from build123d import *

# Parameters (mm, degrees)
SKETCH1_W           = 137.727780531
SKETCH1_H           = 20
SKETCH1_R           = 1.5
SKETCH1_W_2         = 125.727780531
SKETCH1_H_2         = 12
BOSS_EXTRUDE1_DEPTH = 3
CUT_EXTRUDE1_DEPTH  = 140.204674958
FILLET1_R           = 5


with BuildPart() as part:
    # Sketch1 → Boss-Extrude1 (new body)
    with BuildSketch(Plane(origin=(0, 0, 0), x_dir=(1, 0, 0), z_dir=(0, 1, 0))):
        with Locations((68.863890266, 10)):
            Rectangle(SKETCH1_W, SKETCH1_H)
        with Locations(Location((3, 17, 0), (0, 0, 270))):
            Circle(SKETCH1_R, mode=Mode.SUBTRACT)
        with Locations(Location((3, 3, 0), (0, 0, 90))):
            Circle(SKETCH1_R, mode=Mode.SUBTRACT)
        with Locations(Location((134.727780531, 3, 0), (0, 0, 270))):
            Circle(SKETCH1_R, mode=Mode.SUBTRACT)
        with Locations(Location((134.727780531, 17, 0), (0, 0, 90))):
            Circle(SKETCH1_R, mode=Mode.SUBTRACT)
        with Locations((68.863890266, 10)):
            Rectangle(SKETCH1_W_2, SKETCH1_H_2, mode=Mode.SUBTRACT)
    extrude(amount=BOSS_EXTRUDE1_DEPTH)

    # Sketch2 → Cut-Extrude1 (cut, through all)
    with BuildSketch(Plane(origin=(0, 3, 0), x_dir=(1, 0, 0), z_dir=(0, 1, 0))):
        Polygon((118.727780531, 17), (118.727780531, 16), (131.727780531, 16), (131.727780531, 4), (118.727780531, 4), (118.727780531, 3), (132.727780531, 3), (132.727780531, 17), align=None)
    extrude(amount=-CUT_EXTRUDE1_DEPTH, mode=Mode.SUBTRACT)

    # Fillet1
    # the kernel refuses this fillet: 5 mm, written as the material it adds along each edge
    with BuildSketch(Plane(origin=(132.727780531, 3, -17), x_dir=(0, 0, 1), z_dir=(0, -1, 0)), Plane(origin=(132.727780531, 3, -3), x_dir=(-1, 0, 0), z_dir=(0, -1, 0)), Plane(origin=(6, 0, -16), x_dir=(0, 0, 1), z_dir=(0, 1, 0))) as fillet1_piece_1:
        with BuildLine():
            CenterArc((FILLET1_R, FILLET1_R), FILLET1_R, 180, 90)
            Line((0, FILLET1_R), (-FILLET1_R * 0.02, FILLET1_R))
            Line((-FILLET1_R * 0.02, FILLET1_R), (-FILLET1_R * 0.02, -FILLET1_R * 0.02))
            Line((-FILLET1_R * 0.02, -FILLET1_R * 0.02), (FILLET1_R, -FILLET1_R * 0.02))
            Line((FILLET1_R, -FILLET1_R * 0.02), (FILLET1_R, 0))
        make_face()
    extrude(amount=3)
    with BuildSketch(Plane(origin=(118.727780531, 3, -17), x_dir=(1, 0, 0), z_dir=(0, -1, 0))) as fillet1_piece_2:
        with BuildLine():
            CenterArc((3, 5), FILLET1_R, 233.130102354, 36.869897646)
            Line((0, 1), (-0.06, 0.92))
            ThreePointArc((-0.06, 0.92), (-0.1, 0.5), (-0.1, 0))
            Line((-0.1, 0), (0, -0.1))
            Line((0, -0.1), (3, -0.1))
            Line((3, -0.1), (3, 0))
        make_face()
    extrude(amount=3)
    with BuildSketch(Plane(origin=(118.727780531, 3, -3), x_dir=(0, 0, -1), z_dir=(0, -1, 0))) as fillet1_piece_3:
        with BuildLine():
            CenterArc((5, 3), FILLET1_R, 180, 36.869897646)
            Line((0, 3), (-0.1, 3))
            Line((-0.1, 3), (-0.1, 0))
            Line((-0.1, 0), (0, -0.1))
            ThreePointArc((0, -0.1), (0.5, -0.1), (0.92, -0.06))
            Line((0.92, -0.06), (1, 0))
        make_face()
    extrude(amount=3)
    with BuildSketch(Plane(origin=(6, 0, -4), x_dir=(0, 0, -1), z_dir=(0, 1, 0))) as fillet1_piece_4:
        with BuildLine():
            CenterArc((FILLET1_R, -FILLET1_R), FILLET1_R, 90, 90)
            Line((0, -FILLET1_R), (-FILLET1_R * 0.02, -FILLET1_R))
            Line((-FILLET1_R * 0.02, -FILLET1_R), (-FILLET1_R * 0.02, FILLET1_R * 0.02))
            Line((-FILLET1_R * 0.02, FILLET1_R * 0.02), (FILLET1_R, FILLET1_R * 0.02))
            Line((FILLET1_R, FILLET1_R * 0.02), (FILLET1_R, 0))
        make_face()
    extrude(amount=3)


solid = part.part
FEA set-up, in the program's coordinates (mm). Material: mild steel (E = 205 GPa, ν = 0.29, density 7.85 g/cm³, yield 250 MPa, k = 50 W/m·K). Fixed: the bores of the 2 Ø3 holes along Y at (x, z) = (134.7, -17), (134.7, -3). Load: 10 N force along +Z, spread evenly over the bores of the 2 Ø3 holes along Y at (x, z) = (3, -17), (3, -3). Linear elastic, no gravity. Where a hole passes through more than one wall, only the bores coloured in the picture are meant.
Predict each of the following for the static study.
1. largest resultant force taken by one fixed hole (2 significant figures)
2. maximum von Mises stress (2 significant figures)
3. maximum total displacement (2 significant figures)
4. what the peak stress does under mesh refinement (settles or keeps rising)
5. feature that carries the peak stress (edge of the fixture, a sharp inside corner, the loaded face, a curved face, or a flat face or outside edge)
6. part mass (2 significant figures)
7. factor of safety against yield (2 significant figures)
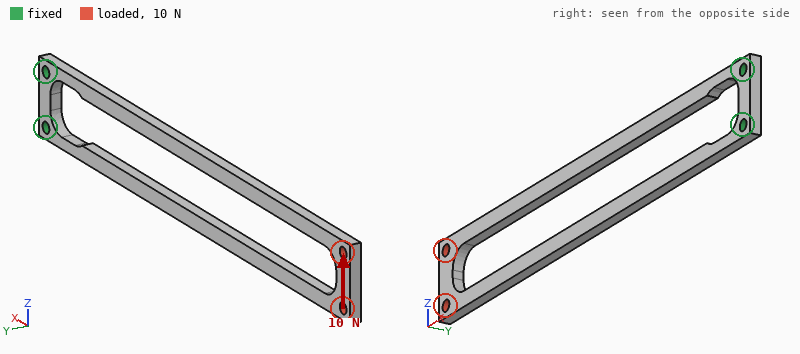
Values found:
57 N
59 MPa
0.32 mm
settles
a flat face or outside edge
28 g
4.2
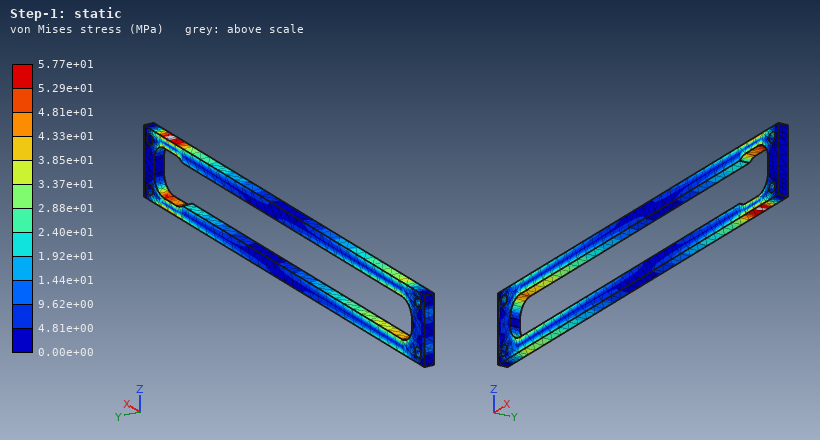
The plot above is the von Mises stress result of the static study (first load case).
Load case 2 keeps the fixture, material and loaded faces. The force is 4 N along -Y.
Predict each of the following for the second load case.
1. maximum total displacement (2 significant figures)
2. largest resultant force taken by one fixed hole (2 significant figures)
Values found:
0.89 mm
2.0 N
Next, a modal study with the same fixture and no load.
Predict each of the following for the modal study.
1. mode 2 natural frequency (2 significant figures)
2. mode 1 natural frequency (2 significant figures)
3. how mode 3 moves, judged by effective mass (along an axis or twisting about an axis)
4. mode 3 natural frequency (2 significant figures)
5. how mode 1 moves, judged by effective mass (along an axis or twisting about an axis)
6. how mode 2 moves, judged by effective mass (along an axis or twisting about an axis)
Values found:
250 Hz
120 Hz
twisting about X
720 Hz
along Y
along Z
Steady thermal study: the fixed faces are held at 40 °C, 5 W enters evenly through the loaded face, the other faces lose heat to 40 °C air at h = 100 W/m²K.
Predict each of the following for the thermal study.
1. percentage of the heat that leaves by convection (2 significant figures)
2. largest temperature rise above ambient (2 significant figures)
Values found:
100 %
60 K
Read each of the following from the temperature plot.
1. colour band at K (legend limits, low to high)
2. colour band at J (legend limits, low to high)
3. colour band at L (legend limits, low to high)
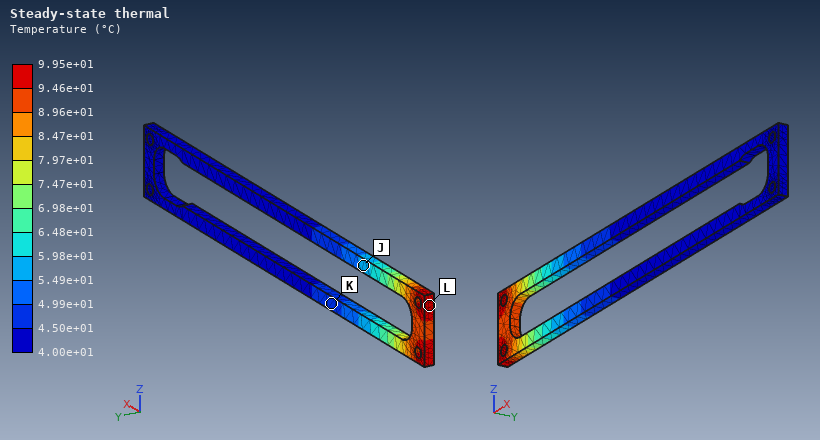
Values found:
4.50e+01 to 4.99e+01 °C
5.49e+01 to 5.98e+01 °C
9.46e+01 to 9.95e+01 °C
